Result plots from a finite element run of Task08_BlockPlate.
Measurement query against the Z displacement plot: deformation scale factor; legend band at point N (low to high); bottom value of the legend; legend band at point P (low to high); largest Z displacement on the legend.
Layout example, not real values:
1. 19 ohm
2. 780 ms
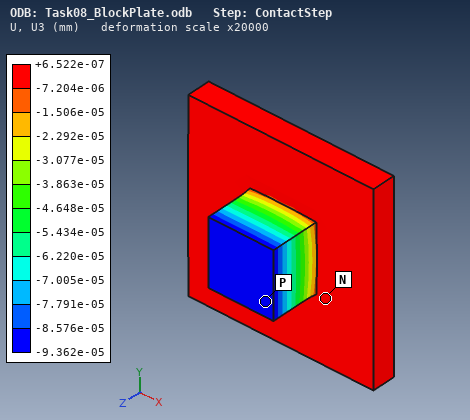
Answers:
1. 20000
2. -7.204e-06 to +6.522e-07 mm
3. -9.362e-05 mm
4. -9.362e-05 to -8.576e-05 mm
5. +6.522e-07 mm
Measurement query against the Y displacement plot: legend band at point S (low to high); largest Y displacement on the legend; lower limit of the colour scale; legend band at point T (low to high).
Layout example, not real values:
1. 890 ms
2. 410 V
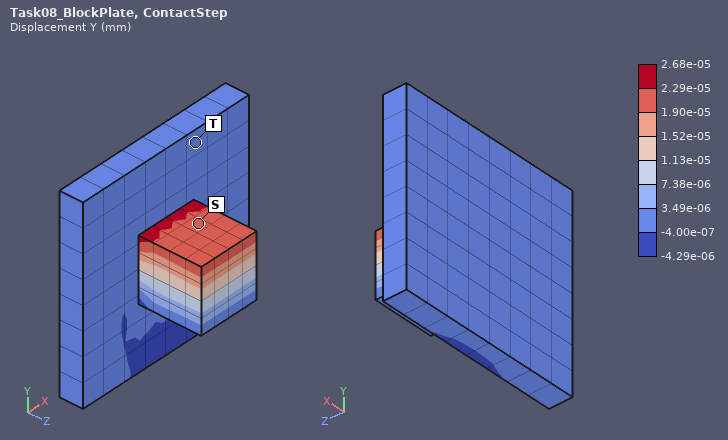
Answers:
1. 1.90e-05 to 2.29e-05 mm
2. 2.68e-05 mm
3. -4.29e-06 mm
4. -4.00e-07 to 3.49e-06 mm
